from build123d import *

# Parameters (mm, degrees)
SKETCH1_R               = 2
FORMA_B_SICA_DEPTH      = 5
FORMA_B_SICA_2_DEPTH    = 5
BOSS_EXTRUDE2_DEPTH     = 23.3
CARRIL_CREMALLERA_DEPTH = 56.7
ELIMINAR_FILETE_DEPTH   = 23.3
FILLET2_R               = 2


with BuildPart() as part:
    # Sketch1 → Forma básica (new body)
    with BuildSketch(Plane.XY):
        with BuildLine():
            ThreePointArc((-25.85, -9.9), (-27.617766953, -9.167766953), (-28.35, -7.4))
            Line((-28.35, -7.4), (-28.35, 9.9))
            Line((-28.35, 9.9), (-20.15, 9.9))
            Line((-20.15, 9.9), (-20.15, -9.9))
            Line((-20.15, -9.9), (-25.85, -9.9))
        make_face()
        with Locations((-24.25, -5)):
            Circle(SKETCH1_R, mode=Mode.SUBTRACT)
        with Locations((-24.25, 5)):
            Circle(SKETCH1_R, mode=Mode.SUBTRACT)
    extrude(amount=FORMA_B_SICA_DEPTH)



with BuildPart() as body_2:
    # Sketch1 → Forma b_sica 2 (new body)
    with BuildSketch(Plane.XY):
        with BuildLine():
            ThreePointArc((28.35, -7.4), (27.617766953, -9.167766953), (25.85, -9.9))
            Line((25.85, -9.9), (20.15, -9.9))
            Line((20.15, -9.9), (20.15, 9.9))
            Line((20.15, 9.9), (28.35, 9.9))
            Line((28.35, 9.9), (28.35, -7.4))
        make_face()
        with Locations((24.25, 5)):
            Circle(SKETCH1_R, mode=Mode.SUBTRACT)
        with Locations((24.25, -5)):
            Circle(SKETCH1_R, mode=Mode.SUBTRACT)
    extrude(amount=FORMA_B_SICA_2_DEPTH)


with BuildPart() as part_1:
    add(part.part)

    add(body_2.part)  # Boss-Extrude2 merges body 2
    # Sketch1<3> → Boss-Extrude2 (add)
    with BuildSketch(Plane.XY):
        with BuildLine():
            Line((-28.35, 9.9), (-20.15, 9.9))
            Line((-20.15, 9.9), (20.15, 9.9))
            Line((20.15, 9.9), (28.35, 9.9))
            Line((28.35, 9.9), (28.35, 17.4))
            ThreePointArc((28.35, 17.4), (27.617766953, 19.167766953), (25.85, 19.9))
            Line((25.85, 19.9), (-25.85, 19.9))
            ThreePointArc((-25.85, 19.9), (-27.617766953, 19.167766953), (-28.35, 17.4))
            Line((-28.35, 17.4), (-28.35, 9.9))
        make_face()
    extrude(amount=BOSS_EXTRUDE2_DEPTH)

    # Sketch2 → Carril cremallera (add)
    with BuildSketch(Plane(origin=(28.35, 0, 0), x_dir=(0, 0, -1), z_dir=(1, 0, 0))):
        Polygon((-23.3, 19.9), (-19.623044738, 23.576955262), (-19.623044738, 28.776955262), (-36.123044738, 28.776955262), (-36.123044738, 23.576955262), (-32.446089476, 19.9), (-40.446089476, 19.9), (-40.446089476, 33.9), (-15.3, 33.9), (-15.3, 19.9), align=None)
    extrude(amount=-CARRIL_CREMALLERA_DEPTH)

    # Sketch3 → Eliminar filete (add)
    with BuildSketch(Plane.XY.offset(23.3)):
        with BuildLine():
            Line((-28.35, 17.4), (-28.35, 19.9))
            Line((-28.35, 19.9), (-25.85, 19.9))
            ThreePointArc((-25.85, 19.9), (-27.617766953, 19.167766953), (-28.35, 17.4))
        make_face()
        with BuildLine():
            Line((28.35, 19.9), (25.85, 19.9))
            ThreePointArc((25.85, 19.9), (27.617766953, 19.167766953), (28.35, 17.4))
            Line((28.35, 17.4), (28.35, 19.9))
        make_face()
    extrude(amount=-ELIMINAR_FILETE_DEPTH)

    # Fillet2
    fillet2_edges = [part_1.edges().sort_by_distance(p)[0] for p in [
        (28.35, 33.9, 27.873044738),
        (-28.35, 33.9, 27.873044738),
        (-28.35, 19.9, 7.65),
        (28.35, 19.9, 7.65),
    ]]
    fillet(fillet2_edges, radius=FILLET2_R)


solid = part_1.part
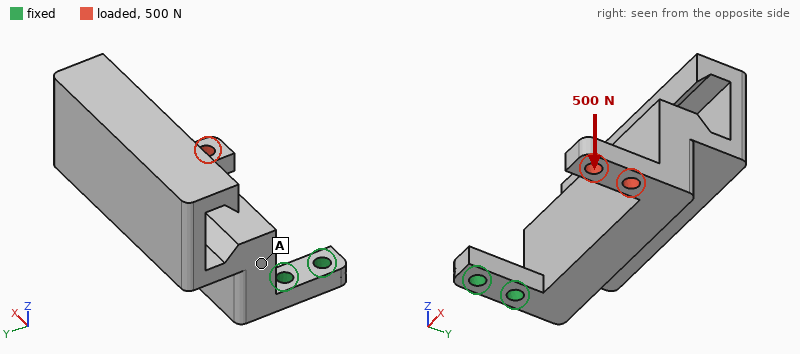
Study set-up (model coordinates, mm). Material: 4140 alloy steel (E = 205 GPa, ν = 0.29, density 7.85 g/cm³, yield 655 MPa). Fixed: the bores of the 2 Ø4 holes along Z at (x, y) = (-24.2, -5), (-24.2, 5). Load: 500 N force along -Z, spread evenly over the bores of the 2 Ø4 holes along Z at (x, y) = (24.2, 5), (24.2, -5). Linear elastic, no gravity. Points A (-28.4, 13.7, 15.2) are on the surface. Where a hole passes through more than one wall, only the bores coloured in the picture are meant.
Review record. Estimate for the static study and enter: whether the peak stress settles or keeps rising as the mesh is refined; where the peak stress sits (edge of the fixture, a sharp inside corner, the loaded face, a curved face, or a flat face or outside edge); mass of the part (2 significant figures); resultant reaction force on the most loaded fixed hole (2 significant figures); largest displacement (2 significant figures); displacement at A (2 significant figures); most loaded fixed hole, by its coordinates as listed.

keeps rising
edge of the fixture
210 g
480 N
0.48 mm
0.097 mm
(-24.2, 5)
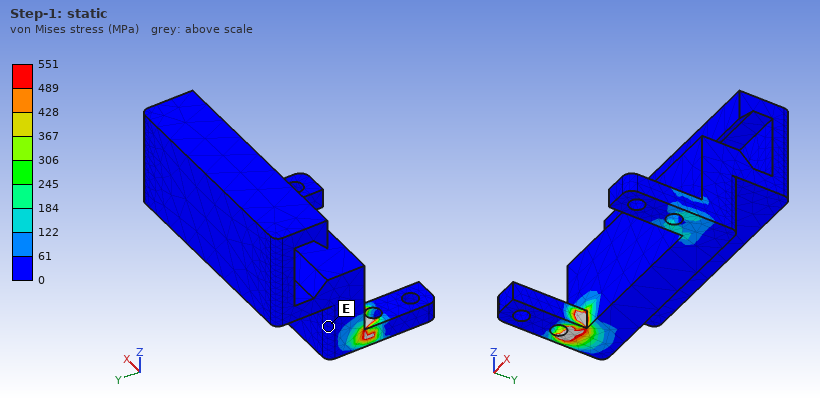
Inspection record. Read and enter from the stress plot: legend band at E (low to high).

0 to 61 MPa
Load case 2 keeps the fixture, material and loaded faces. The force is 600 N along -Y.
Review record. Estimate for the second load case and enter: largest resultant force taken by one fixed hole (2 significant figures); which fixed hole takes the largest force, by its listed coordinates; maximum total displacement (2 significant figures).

840 N
(-24.2, 5)
0.36 mm
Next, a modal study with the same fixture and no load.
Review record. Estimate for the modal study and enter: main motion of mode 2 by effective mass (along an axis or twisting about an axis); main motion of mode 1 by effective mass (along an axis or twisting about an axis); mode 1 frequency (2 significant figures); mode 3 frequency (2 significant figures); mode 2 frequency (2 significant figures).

along Y
along Z
540 Hz
1200 Hz
610 Hz
